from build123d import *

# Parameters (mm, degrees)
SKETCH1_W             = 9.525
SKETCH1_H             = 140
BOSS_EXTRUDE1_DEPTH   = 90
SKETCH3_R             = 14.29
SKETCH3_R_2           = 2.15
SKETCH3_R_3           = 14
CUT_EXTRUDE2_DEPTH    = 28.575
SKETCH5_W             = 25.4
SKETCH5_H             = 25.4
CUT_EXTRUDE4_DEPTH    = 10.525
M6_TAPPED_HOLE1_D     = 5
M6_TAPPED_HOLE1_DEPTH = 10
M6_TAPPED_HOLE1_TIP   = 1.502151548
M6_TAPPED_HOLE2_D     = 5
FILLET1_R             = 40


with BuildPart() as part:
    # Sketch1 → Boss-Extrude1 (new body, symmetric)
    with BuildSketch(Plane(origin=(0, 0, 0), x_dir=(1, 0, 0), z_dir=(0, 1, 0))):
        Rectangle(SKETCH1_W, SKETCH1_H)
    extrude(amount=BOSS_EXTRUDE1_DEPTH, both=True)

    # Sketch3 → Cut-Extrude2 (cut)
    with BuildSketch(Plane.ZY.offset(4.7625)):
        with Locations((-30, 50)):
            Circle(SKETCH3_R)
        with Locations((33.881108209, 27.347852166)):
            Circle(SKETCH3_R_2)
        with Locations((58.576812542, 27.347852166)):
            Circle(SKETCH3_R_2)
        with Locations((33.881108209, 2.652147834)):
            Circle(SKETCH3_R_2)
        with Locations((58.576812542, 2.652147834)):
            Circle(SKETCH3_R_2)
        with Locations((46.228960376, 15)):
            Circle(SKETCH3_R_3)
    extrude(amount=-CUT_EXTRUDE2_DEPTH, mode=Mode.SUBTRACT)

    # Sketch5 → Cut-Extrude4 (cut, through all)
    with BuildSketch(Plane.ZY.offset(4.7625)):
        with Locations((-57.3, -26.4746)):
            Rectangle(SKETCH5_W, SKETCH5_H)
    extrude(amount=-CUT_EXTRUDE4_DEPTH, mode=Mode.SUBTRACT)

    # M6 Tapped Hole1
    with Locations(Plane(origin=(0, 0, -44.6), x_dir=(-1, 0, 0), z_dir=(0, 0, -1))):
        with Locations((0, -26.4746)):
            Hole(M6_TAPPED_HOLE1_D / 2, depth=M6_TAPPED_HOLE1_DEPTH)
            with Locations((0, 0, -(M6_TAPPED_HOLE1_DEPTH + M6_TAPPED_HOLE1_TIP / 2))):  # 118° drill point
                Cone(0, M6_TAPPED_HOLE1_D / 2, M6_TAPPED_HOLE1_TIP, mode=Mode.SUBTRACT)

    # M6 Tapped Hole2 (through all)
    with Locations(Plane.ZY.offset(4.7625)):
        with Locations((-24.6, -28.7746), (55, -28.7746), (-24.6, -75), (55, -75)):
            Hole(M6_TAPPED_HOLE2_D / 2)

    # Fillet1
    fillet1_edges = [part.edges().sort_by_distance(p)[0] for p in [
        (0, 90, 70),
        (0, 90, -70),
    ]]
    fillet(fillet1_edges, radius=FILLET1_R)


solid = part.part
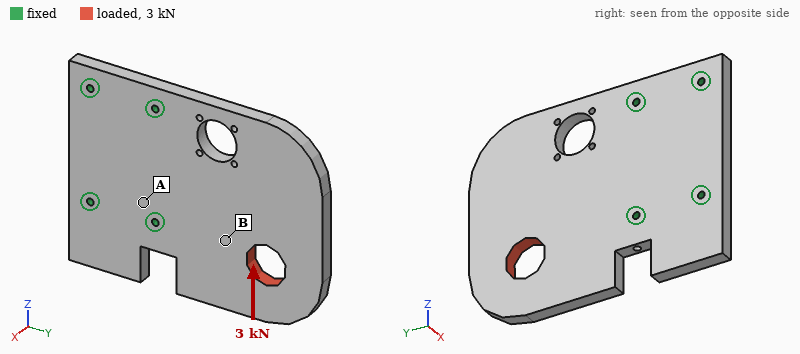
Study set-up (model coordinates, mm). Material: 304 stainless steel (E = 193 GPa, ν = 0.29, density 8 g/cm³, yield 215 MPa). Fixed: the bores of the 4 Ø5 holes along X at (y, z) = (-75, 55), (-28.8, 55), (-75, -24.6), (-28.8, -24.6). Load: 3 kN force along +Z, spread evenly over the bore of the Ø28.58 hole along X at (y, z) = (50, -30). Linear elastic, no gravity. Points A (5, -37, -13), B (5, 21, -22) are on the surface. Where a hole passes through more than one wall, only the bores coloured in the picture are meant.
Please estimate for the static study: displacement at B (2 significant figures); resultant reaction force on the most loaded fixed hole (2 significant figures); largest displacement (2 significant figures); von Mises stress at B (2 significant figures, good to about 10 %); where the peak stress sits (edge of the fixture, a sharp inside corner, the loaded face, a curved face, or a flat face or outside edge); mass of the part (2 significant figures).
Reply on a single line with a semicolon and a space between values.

5.4 µm; 2.8 kN; 12 µm; 8.3 MPa; a curved face; 1.7 kg
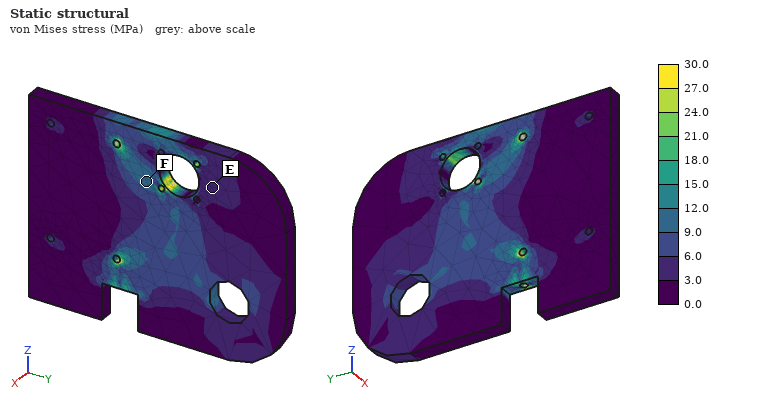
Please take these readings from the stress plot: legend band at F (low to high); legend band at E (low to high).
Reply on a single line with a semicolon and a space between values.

9.0 to 12.0 MPa; 3.0 to 6.0 MPa
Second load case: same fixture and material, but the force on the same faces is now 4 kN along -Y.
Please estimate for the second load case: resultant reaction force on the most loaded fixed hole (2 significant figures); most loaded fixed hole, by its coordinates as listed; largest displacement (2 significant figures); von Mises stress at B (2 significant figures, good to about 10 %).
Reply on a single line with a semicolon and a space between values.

3.2 kN; (-28.8, -24.6); 7.4 µm; 7.4 MPa
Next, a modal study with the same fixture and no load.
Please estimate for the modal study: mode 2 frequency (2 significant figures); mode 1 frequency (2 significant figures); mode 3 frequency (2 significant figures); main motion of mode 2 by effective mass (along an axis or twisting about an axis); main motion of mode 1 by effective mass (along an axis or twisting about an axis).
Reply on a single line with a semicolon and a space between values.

1100 Hz; 480 Hz; 2500 Hz; twisting about Y; along X
